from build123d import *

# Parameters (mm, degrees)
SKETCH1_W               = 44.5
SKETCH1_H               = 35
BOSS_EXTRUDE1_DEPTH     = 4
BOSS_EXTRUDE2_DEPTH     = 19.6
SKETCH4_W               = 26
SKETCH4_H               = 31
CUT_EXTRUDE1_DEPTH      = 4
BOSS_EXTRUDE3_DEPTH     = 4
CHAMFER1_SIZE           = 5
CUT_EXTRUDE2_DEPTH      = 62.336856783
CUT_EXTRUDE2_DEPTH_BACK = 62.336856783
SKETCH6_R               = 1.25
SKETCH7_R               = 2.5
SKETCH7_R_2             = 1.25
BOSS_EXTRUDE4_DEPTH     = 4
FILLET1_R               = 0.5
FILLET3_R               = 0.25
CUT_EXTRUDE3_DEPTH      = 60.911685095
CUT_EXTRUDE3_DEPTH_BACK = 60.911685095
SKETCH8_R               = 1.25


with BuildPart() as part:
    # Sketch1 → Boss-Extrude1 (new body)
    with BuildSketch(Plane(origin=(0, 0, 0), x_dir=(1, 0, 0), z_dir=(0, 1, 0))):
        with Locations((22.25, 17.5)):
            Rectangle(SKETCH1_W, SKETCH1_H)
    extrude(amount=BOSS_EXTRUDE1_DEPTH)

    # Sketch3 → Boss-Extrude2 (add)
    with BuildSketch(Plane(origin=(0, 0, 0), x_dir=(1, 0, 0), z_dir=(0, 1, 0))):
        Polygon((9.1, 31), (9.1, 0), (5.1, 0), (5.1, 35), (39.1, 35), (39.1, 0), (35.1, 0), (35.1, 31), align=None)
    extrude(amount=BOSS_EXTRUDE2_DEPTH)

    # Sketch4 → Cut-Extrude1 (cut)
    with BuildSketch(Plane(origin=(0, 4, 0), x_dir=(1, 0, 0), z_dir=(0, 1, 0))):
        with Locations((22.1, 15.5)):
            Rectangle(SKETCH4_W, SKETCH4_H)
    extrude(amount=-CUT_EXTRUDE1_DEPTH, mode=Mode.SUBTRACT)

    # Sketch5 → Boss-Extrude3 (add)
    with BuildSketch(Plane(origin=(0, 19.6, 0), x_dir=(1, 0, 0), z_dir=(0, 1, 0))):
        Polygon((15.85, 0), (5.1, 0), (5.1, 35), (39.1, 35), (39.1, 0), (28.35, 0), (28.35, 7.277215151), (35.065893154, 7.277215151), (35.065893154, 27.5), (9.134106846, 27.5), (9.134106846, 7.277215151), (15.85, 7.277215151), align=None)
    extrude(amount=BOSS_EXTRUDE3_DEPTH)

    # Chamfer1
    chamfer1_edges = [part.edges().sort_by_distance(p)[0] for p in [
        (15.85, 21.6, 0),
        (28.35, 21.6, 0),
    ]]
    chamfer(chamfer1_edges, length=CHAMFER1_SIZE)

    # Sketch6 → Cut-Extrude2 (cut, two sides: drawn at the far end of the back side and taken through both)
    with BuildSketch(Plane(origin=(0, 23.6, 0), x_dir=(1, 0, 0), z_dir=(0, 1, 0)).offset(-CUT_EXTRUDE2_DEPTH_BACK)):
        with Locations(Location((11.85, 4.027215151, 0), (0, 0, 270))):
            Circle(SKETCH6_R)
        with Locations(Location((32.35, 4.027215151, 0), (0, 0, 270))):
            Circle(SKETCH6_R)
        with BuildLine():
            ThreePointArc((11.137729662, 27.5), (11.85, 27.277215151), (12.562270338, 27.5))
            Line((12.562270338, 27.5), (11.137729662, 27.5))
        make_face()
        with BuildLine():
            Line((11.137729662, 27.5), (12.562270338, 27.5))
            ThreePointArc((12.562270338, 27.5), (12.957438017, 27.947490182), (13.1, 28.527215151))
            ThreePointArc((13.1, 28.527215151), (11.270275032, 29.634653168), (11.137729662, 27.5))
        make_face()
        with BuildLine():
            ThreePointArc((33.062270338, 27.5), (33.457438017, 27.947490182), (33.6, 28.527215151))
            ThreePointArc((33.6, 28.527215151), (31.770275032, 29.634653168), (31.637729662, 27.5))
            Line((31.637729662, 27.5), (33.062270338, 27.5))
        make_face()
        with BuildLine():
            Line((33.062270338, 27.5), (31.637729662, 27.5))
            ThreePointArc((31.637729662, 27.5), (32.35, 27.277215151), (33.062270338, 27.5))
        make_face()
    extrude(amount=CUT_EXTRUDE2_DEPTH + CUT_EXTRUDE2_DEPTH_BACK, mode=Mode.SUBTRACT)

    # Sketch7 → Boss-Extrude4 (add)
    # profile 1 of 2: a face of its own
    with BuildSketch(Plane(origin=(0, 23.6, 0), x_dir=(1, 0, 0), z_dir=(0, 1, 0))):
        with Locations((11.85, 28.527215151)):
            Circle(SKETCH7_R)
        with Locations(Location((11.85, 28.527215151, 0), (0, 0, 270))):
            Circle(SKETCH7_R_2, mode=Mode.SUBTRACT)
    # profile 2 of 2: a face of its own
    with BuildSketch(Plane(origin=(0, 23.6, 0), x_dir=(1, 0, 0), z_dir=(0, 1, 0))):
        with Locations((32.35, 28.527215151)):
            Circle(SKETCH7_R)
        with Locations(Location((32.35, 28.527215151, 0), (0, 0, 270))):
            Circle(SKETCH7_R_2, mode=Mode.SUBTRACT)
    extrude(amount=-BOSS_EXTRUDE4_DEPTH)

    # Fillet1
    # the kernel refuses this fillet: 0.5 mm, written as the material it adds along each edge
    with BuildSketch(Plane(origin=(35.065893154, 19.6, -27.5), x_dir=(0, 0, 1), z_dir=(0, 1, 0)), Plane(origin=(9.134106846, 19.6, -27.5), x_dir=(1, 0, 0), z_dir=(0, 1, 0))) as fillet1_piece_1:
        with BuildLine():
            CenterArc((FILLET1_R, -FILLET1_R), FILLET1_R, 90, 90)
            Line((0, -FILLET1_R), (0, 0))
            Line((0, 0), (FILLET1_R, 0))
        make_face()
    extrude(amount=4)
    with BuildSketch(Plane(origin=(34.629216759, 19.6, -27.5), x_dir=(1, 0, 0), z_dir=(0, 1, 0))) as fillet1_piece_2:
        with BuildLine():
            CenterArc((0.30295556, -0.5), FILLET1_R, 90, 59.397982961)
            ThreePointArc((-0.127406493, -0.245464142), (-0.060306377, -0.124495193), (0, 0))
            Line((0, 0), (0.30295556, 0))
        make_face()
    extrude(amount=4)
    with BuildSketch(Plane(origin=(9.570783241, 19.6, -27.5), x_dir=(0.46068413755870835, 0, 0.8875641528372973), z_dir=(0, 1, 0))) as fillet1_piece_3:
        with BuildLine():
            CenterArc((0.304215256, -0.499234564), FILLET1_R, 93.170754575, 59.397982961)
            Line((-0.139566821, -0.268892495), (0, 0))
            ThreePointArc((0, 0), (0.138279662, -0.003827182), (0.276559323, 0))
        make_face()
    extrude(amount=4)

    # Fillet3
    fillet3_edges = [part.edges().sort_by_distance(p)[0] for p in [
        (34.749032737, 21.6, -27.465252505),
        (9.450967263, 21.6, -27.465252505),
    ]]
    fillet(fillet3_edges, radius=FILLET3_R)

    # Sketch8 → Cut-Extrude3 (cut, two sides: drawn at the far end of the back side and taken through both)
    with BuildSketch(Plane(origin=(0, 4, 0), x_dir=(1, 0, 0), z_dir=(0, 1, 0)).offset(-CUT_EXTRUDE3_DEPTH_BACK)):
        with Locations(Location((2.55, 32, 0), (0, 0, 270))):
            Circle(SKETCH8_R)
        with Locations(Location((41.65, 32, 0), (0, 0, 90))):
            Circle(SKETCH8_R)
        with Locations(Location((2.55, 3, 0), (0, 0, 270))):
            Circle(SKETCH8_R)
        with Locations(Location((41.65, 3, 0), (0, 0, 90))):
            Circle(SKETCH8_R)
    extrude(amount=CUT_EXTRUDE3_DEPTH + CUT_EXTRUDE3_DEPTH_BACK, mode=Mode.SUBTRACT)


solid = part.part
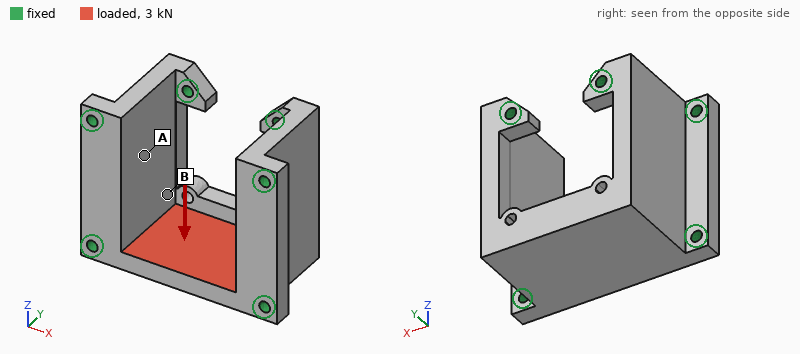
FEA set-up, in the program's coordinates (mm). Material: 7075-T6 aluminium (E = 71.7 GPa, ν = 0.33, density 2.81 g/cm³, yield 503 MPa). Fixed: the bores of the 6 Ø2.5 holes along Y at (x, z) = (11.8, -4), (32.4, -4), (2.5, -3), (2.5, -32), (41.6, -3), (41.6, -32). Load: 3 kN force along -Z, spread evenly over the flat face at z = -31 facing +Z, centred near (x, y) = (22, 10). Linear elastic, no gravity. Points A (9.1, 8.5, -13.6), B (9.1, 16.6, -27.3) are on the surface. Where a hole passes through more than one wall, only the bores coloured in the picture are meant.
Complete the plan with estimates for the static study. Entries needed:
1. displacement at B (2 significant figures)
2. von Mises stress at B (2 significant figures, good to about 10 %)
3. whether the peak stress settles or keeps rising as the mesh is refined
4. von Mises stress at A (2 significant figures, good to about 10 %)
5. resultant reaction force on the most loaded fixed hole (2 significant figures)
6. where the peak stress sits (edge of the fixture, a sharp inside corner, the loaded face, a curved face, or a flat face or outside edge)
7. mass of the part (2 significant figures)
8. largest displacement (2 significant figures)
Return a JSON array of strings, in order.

["13 µm", "44 MPa", "keeps rising", "13 MPa", "790 N", "edge of the fixture", "31 g", "58 µm"]
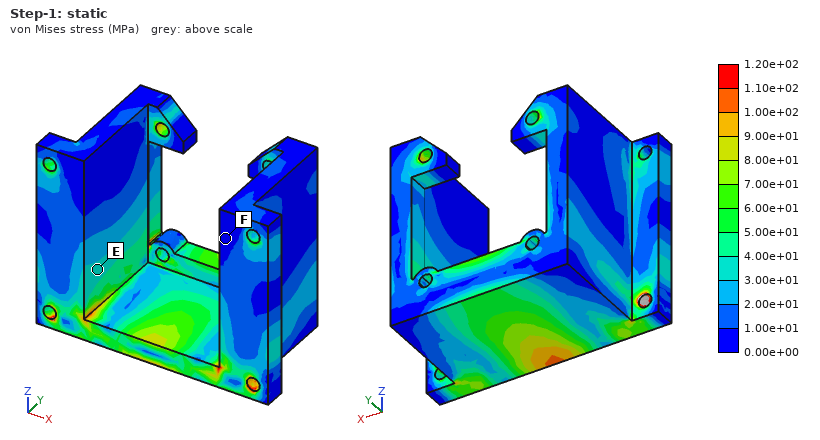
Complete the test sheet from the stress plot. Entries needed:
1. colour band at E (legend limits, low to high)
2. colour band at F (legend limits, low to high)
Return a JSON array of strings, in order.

["3.00e+01 to 4.00e+01 MPa", "0.00e+00 to 1.00e+01 MPa"]
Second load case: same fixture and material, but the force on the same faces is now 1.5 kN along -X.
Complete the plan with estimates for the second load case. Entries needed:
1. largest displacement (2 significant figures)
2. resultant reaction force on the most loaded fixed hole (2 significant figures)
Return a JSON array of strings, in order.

["7.7 µm", "790 N"]
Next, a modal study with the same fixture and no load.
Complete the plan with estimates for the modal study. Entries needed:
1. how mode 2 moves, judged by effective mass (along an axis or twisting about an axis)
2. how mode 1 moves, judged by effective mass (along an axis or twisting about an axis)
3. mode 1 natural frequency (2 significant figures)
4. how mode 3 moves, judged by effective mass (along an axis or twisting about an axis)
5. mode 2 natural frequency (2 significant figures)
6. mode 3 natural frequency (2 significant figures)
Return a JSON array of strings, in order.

["along X", "along Z", "14 kHz", "along Y", "18 kHz", "19 kHz"]
